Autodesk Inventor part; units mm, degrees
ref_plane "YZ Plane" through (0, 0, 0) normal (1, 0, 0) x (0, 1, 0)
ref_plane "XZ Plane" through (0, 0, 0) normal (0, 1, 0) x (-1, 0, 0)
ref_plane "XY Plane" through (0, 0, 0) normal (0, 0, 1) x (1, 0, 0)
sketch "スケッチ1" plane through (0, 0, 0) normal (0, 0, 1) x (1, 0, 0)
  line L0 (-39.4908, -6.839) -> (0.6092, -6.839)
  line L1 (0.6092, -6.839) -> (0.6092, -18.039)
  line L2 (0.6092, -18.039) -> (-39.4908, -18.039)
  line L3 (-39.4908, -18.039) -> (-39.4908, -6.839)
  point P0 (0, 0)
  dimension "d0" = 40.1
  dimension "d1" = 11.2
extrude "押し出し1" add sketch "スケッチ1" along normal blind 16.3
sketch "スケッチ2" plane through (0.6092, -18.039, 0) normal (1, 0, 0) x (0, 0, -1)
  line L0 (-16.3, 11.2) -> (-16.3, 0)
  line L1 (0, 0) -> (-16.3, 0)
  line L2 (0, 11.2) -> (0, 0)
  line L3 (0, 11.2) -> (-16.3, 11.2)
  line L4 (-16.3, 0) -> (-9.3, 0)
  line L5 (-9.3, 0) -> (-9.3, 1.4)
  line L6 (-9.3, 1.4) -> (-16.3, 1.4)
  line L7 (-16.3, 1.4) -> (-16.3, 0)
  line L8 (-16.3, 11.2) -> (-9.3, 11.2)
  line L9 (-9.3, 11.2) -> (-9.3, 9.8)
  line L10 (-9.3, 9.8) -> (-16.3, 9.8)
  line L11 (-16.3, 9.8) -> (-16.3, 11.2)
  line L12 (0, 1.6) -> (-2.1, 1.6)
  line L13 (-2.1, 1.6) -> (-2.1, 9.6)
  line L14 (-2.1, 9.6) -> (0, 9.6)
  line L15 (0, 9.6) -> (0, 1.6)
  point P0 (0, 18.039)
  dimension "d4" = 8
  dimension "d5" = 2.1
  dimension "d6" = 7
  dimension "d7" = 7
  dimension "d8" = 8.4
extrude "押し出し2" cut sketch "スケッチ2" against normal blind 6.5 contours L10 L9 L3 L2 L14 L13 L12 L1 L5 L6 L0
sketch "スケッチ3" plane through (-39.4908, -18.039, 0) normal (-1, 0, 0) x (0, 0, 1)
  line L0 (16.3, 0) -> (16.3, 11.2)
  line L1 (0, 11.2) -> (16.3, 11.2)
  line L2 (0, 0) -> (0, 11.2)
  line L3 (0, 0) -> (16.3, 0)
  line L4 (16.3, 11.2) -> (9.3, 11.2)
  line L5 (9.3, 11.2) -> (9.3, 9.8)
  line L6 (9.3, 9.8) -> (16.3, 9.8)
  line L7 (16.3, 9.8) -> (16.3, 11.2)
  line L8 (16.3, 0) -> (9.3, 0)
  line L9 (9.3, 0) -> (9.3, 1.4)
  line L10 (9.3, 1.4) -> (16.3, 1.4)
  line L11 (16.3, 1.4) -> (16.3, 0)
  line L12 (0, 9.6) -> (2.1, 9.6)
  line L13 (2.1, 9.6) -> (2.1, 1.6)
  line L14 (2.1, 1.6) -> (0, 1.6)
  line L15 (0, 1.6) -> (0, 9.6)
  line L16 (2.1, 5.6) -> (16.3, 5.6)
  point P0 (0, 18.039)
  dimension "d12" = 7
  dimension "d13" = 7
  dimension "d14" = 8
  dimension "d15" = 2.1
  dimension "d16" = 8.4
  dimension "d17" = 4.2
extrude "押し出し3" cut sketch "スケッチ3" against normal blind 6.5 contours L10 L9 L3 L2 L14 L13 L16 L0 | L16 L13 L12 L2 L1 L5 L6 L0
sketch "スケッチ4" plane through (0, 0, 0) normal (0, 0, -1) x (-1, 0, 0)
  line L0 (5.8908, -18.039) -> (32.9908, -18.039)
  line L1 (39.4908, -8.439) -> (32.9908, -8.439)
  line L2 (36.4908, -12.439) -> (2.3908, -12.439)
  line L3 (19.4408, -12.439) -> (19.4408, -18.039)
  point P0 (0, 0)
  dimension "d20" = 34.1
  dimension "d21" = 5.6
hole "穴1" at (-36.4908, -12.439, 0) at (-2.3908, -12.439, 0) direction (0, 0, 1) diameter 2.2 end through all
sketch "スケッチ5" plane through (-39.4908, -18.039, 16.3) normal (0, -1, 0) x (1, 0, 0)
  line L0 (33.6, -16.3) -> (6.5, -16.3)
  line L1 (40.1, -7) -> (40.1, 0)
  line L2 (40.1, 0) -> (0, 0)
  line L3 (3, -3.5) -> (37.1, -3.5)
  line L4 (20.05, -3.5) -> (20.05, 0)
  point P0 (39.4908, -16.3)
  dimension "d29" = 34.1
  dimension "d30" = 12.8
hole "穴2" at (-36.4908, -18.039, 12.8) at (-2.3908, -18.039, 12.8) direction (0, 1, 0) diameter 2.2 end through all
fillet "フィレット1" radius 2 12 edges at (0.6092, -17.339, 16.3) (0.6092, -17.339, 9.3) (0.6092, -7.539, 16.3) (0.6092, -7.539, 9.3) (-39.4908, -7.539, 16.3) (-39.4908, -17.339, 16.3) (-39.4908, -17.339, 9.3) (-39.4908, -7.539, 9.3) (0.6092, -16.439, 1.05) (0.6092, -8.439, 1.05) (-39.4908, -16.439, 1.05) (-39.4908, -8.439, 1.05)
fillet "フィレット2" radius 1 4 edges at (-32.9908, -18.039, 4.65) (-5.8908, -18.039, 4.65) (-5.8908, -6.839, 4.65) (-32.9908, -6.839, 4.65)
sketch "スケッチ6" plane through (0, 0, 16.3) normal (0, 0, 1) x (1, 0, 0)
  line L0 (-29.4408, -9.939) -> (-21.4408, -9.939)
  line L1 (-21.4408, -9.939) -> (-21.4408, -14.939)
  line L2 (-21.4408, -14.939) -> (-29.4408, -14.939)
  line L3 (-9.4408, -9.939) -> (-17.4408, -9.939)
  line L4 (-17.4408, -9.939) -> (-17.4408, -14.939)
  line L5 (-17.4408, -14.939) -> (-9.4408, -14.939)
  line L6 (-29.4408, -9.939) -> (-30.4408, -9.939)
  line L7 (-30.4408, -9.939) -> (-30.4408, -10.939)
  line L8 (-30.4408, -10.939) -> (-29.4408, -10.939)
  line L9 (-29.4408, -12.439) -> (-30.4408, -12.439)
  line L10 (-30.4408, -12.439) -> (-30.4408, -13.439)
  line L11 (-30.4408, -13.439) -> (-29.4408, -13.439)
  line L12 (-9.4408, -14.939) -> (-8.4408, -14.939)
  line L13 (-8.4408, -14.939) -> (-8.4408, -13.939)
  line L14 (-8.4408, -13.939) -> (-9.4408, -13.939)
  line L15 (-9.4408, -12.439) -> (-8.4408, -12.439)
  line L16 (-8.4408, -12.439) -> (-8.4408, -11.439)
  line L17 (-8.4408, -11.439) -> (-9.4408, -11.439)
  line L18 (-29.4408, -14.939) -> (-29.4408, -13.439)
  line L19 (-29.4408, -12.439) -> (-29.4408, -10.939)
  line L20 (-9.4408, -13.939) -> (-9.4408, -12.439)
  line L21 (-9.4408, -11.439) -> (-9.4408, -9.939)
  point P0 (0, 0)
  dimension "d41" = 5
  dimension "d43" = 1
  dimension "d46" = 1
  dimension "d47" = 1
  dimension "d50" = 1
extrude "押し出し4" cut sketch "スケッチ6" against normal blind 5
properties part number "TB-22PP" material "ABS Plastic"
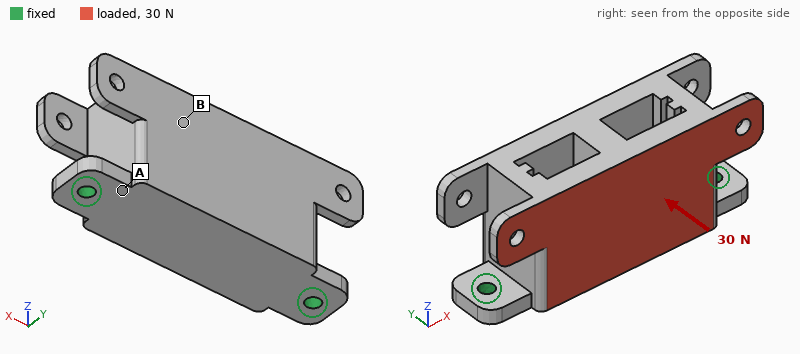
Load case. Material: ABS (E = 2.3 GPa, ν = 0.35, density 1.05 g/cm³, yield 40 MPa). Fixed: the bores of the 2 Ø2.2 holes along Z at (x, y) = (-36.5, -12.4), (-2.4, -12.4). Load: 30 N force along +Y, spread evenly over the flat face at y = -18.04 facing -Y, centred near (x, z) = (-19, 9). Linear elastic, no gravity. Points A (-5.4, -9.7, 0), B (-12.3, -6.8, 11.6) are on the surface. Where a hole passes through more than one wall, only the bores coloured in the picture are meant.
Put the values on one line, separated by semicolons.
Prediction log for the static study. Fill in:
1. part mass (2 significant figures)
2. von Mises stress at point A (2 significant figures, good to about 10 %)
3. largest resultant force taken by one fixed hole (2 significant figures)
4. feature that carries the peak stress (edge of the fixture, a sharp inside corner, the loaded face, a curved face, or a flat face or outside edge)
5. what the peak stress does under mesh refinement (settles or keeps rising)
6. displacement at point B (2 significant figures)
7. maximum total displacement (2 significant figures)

5.2 g; 7.6 MPa; 15 N; edge of the fixture; keeps rising; 0.23 mm; 0.33 mm
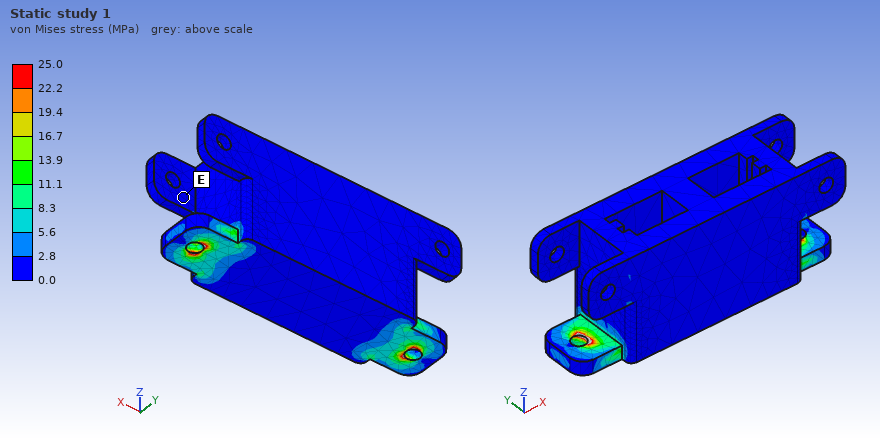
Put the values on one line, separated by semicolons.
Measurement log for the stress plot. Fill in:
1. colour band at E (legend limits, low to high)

0.0 to 2.8 MPa
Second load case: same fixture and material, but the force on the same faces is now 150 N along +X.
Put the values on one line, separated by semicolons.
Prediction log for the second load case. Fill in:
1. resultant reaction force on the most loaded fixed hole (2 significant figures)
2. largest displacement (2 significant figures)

89 N; 0.11 mm
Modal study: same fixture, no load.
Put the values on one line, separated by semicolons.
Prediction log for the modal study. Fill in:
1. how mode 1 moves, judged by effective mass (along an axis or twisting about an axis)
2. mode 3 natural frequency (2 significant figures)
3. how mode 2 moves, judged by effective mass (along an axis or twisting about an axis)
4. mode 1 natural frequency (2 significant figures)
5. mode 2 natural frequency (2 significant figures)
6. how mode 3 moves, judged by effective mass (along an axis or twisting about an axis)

along Y; 4200 Hz; along Z; 890 Hz; 3400 Hz; along X
